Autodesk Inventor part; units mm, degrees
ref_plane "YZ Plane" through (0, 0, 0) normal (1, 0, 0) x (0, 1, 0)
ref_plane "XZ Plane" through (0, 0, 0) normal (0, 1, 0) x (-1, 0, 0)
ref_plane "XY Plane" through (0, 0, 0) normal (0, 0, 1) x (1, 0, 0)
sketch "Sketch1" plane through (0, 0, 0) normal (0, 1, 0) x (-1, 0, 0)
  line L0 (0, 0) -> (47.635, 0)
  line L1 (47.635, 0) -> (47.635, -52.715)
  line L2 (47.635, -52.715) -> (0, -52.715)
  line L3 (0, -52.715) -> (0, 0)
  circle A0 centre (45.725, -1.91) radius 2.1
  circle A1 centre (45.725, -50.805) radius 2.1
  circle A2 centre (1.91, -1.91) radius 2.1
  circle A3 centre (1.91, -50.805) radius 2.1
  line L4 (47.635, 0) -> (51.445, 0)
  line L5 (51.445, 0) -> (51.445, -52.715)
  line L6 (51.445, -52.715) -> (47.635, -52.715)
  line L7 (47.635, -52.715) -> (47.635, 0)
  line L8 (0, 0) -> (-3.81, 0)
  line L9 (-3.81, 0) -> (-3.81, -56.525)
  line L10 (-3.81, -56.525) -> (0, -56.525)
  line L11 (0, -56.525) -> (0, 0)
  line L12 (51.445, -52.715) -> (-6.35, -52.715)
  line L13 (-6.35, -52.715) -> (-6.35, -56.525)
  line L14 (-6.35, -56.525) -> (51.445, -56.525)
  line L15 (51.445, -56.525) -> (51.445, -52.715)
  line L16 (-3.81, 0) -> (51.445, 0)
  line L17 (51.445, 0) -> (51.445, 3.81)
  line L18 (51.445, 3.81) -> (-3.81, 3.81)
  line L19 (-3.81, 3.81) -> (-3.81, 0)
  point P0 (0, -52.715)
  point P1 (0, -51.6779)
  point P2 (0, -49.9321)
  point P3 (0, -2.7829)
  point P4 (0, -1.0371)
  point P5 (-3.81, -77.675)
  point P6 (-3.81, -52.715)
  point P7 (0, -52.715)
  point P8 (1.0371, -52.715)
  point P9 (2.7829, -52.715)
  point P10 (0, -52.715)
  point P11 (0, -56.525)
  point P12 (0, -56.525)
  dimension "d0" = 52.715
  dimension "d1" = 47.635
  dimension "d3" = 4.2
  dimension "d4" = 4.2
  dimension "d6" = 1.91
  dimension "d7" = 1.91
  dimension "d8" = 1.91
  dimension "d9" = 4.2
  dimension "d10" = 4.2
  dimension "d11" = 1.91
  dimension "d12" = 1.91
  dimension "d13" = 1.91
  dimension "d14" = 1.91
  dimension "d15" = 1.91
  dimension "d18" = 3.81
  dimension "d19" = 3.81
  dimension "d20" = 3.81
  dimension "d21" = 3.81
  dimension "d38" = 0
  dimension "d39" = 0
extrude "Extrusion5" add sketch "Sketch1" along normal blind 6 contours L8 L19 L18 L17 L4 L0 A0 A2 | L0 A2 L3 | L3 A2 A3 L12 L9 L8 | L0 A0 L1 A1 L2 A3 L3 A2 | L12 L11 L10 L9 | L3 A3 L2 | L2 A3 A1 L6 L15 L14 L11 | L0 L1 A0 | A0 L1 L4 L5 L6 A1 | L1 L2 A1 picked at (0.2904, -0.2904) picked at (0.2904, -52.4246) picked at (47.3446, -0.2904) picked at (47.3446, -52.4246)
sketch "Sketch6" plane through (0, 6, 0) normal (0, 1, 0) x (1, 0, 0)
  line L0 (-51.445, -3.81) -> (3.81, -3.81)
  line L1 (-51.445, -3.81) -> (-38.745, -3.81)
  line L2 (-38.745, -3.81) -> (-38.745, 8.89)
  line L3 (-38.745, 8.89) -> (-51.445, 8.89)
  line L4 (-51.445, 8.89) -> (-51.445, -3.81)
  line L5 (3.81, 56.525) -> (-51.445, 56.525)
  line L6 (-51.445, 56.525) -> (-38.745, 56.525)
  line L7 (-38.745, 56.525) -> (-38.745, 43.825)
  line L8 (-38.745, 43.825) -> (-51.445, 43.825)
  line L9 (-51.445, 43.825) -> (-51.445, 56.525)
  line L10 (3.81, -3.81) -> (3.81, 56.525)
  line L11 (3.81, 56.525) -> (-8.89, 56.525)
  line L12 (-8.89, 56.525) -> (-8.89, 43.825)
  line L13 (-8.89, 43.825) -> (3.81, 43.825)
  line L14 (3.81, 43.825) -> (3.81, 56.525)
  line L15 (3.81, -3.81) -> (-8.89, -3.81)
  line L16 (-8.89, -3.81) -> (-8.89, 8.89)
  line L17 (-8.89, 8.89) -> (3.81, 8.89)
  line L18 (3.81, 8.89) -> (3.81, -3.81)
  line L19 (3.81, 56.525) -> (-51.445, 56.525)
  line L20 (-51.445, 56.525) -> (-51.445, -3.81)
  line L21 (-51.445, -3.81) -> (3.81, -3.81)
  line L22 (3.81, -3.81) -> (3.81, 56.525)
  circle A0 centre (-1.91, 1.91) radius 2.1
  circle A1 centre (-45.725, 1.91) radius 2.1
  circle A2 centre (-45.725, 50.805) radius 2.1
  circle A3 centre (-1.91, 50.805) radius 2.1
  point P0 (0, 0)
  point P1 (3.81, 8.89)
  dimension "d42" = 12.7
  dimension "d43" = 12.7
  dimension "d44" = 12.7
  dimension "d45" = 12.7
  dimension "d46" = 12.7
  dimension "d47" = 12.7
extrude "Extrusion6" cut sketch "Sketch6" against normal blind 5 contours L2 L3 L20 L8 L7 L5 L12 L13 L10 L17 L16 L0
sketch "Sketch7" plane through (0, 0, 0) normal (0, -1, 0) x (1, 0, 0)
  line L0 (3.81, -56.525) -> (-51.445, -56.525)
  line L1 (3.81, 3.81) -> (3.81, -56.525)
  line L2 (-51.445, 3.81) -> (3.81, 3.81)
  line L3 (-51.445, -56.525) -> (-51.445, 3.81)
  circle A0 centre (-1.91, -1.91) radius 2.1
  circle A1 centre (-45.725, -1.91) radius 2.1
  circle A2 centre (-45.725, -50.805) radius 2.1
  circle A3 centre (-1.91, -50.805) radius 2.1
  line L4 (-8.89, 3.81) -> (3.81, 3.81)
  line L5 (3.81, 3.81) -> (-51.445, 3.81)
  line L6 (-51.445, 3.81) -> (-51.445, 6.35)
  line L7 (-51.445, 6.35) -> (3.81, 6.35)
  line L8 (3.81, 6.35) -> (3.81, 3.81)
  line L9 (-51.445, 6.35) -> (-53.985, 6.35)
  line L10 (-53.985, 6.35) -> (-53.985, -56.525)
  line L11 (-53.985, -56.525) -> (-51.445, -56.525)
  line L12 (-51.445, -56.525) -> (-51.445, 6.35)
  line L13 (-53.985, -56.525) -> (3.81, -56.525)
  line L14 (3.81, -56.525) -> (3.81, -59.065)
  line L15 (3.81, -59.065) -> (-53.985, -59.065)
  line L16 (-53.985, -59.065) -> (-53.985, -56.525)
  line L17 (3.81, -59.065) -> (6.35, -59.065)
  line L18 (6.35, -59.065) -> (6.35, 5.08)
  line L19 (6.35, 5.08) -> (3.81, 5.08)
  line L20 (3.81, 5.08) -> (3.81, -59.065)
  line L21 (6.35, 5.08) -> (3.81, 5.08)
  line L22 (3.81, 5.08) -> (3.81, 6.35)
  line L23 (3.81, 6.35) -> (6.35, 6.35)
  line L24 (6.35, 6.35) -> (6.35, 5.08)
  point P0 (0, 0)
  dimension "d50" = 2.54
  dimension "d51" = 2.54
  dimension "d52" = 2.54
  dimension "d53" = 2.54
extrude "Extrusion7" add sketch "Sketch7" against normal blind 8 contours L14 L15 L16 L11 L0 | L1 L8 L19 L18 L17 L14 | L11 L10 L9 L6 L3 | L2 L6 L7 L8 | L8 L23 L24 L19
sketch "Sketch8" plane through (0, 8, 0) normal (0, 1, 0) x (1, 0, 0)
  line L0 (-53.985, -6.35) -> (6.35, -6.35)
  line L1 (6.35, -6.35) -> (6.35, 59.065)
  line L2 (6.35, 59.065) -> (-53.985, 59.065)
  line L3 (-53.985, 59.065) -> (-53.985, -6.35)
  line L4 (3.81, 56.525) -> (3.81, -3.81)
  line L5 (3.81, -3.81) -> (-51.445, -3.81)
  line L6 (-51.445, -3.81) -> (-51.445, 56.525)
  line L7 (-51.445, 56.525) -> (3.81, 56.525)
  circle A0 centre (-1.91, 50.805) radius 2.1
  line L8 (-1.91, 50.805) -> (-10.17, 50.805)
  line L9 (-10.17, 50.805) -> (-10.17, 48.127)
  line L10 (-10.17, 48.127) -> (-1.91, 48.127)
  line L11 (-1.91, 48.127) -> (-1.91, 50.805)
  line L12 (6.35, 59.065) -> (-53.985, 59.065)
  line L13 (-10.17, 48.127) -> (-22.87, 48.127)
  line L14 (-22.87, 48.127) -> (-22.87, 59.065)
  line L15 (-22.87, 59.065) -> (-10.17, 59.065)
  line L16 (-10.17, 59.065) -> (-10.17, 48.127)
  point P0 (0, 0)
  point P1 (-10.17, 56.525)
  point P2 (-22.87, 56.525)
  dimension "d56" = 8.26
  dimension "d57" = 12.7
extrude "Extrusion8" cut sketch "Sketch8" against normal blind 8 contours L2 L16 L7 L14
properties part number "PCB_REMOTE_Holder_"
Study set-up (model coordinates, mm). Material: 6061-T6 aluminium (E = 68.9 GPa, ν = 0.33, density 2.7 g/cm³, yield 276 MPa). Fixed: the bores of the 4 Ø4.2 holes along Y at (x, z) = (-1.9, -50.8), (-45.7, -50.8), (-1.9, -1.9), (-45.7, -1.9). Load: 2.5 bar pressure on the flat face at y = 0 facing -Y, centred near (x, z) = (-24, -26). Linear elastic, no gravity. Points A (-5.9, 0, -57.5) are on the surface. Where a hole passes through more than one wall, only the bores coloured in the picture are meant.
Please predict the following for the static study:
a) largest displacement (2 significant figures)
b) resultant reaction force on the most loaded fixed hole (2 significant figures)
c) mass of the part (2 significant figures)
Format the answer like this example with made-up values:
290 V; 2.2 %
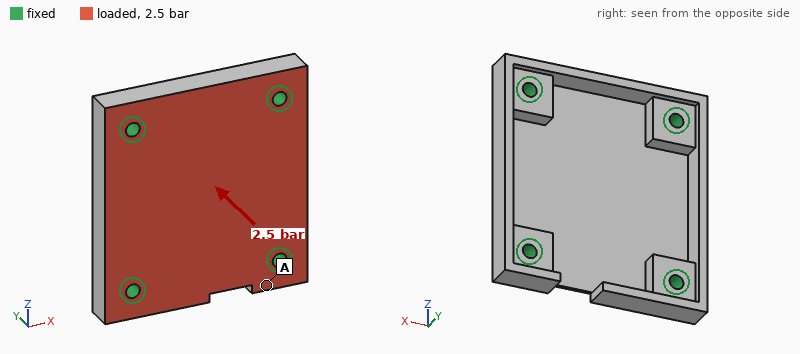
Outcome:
0.32 mm; 290 N; 29 g
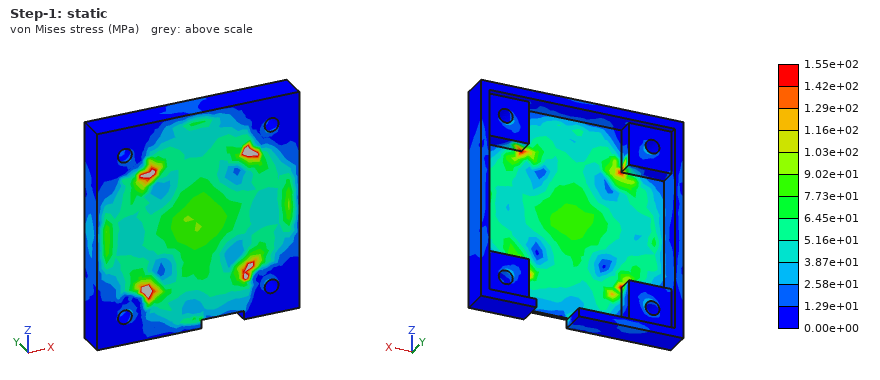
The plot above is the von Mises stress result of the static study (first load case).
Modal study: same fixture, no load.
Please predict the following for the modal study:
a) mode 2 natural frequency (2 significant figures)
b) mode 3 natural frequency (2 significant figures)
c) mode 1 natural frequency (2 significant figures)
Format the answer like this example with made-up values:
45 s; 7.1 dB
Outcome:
6700 Hz; 6800 Hz; 3500 Hz
